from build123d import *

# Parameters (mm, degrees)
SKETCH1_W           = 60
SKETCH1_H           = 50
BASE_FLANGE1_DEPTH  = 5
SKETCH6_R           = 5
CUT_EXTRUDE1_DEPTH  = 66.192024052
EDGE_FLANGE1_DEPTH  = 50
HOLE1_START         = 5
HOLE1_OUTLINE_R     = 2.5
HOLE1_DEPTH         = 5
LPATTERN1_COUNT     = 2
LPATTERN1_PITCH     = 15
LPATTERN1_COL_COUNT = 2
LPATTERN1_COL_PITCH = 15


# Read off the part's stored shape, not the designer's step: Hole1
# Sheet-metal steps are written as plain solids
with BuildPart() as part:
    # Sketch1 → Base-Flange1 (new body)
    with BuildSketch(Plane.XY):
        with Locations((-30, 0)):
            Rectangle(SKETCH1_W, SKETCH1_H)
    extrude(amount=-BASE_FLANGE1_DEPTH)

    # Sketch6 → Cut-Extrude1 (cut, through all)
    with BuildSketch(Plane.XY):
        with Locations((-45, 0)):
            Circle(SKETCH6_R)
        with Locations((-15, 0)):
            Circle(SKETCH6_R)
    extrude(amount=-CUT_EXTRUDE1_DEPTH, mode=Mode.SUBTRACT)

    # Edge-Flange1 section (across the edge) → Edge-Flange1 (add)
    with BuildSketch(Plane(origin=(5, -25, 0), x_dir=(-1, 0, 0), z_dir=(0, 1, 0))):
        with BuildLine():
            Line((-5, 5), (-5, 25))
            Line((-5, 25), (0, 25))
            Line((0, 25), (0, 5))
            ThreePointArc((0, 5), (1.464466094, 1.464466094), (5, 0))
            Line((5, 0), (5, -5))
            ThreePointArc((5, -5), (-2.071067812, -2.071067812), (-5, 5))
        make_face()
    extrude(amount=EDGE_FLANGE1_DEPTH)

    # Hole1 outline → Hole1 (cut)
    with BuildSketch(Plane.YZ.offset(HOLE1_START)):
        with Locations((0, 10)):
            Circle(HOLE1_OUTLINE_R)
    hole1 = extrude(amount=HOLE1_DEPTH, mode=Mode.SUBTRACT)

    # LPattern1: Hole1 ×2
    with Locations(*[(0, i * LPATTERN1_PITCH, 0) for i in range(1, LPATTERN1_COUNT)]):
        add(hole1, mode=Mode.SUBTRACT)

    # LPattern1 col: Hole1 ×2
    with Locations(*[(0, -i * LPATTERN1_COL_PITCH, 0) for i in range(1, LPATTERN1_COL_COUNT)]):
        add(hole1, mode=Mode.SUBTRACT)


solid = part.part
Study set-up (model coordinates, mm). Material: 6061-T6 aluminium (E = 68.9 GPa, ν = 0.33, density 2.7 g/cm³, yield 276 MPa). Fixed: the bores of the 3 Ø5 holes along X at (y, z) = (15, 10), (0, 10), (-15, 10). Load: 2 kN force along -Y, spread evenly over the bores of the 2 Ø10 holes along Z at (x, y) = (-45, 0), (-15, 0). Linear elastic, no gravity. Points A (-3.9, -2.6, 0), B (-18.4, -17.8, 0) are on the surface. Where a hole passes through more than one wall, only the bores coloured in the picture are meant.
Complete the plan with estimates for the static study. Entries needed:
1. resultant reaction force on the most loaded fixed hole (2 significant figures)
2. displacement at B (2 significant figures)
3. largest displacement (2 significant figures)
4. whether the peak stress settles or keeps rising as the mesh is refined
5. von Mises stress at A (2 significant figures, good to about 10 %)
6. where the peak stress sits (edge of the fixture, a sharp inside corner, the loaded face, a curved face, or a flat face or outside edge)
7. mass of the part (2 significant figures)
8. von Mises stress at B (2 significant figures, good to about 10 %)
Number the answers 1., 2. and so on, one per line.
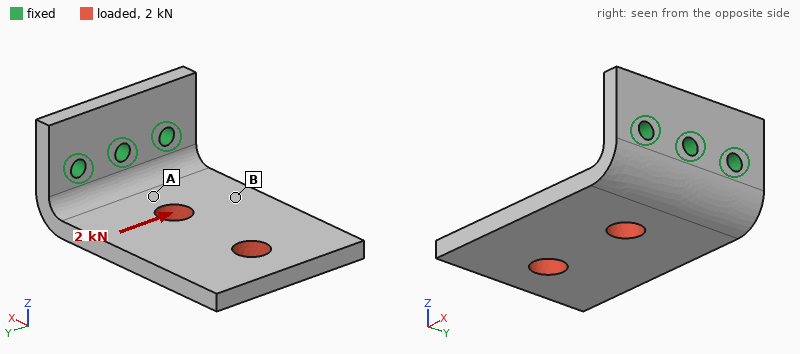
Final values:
1. 2.4 kN
2. 0.14 mm
3. 0.31 mm
4. keeps rising
5. 63 MPa
6. edge of the fixture
7. 59 g
8. 29 MPa
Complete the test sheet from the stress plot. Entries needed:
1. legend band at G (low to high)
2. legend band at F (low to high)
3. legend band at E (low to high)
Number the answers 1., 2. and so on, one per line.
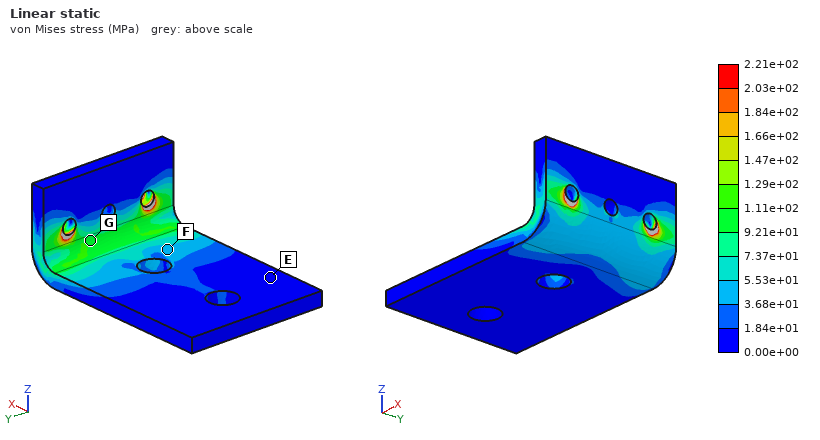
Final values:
1. 9.21e+01 to 1.11e+02 MPa
2. 3.68e+01 to 5.53e+01 MPa
3. 0.00e+00 to 1.84e+01 MPa
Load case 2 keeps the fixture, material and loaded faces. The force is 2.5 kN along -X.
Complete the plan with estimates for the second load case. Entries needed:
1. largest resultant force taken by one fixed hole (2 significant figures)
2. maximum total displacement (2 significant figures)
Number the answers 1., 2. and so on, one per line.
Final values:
1. 850 N
2. 0.34 mm
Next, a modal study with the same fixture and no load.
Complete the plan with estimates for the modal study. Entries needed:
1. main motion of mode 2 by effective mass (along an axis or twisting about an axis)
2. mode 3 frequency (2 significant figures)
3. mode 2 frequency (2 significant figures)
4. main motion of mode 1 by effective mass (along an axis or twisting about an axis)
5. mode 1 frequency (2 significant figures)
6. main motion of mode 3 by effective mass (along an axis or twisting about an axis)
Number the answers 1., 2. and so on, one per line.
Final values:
1. along Y
2. 3100 Hz
3. 2200 Hz
4. along Z
5. 750 Hz
6. along Y
